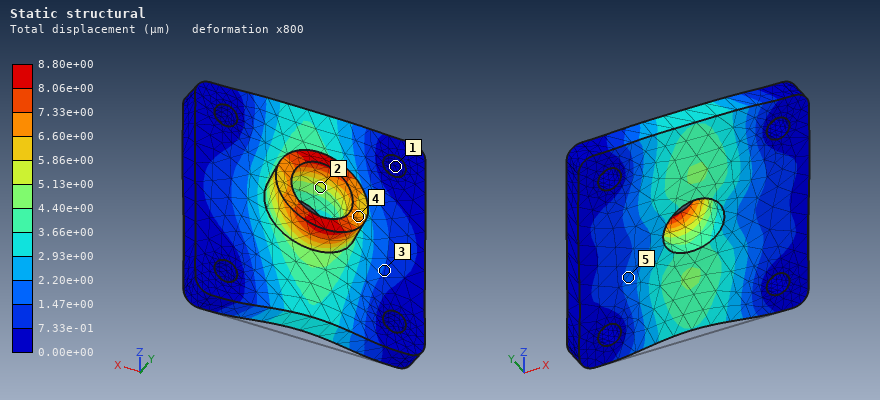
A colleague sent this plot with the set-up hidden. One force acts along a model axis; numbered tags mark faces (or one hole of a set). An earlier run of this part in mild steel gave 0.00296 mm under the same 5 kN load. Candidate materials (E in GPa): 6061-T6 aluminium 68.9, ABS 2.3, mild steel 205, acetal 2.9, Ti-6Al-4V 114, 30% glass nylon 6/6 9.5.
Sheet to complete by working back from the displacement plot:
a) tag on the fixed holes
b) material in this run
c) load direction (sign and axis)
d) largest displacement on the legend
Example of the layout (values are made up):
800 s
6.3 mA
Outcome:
1
6061-T6 aluminium
+Z
8.80e+00 µm
